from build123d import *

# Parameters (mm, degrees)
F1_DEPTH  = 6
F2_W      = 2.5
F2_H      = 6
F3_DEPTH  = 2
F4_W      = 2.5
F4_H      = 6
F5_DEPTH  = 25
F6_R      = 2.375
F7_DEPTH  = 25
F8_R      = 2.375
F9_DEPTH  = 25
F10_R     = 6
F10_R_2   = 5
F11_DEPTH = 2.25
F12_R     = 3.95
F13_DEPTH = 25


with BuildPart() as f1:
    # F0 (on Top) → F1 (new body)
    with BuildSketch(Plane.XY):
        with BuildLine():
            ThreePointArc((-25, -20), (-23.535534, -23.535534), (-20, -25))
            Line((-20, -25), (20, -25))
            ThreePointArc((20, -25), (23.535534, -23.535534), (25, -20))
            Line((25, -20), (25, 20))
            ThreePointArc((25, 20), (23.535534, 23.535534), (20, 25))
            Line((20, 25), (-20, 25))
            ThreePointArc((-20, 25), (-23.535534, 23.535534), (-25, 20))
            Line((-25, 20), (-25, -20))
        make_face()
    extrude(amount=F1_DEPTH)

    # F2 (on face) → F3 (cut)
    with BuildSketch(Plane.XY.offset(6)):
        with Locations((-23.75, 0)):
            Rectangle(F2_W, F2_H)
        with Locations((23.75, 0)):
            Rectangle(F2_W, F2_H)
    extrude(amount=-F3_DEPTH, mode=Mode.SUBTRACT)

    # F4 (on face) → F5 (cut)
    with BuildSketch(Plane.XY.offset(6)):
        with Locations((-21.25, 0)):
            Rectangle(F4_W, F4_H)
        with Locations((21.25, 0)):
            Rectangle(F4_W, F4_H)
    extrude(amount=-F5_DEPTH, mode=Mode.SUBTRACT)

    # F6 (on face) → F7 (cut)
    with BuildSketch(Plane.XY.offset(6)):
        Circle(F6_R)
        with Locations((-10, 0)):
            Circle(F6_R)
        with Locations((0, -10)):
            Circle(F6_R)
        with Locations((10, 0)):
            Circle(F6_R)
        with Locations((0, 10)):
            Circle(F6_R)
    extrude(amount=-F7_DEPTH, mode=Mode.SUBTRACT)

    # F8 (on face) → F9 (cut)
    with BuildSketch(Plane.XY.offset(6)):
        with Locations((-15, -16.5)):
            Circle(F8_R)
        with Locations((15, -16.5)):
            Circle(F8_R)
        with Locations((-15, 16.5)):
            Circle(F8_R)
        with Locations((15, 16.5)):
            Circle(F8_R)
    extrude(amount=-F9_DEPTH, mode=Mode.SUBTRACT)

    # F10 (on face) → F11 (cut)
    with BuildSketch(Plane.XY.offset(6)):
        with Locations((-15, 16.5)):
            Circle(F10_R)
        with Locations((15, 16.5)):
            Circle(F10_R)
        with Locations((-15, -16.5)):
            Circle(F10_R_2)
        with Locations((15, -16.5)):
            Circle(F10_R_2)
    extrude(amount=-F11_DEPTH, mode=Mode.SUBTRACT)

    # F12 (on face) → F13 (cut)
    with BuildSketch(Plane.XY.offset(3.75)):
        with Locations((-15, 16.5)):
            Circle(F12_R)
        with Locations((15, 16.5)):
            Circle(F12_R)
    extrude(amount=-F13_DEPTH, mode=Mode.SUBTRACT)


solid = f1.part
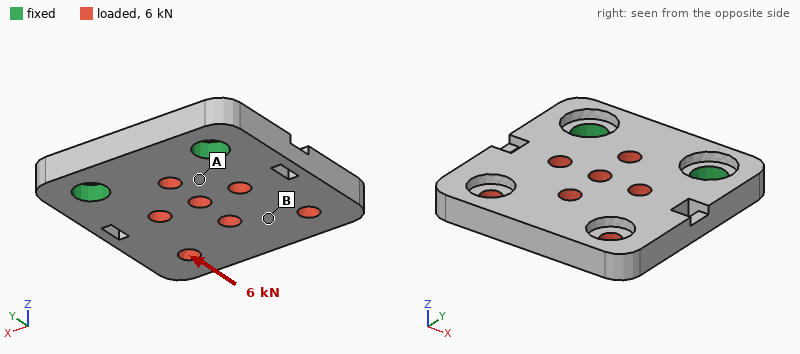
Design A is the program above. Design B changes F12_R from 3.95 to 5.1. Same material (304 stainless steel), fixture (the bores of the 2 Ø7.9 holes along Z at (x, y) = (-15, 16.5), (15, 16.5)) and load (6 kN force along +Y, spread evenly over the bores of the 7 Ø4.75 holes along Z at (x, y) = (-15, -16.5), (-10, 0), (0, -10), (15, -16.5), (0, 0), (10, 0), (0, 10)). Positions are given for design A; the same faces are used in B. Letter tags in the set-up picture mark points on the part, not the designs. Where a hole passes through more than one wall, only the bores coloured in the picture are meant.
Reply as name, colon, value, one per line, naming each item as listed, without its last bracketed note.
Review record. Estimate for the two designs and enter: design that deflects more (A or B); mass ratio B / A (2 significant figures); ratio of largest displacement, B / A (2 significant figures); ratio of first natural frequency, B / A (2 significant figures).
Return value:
design that deflects more: A
mass ratio B / A: 0.98
ratio of largest displacement, B / A: 0.60
ratio of first natural frequency, B / A: 1.1
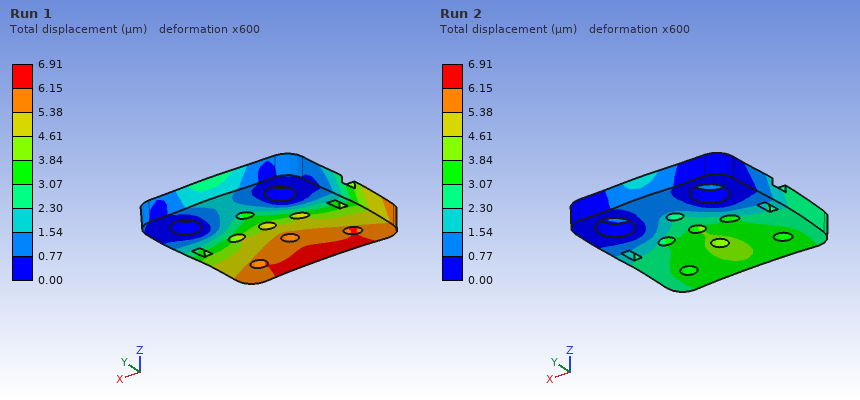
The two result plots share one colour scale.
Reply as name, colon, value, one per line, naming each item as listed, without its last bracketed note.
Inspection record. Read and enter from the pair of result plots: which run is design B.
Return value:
which run is design B: Run 2
